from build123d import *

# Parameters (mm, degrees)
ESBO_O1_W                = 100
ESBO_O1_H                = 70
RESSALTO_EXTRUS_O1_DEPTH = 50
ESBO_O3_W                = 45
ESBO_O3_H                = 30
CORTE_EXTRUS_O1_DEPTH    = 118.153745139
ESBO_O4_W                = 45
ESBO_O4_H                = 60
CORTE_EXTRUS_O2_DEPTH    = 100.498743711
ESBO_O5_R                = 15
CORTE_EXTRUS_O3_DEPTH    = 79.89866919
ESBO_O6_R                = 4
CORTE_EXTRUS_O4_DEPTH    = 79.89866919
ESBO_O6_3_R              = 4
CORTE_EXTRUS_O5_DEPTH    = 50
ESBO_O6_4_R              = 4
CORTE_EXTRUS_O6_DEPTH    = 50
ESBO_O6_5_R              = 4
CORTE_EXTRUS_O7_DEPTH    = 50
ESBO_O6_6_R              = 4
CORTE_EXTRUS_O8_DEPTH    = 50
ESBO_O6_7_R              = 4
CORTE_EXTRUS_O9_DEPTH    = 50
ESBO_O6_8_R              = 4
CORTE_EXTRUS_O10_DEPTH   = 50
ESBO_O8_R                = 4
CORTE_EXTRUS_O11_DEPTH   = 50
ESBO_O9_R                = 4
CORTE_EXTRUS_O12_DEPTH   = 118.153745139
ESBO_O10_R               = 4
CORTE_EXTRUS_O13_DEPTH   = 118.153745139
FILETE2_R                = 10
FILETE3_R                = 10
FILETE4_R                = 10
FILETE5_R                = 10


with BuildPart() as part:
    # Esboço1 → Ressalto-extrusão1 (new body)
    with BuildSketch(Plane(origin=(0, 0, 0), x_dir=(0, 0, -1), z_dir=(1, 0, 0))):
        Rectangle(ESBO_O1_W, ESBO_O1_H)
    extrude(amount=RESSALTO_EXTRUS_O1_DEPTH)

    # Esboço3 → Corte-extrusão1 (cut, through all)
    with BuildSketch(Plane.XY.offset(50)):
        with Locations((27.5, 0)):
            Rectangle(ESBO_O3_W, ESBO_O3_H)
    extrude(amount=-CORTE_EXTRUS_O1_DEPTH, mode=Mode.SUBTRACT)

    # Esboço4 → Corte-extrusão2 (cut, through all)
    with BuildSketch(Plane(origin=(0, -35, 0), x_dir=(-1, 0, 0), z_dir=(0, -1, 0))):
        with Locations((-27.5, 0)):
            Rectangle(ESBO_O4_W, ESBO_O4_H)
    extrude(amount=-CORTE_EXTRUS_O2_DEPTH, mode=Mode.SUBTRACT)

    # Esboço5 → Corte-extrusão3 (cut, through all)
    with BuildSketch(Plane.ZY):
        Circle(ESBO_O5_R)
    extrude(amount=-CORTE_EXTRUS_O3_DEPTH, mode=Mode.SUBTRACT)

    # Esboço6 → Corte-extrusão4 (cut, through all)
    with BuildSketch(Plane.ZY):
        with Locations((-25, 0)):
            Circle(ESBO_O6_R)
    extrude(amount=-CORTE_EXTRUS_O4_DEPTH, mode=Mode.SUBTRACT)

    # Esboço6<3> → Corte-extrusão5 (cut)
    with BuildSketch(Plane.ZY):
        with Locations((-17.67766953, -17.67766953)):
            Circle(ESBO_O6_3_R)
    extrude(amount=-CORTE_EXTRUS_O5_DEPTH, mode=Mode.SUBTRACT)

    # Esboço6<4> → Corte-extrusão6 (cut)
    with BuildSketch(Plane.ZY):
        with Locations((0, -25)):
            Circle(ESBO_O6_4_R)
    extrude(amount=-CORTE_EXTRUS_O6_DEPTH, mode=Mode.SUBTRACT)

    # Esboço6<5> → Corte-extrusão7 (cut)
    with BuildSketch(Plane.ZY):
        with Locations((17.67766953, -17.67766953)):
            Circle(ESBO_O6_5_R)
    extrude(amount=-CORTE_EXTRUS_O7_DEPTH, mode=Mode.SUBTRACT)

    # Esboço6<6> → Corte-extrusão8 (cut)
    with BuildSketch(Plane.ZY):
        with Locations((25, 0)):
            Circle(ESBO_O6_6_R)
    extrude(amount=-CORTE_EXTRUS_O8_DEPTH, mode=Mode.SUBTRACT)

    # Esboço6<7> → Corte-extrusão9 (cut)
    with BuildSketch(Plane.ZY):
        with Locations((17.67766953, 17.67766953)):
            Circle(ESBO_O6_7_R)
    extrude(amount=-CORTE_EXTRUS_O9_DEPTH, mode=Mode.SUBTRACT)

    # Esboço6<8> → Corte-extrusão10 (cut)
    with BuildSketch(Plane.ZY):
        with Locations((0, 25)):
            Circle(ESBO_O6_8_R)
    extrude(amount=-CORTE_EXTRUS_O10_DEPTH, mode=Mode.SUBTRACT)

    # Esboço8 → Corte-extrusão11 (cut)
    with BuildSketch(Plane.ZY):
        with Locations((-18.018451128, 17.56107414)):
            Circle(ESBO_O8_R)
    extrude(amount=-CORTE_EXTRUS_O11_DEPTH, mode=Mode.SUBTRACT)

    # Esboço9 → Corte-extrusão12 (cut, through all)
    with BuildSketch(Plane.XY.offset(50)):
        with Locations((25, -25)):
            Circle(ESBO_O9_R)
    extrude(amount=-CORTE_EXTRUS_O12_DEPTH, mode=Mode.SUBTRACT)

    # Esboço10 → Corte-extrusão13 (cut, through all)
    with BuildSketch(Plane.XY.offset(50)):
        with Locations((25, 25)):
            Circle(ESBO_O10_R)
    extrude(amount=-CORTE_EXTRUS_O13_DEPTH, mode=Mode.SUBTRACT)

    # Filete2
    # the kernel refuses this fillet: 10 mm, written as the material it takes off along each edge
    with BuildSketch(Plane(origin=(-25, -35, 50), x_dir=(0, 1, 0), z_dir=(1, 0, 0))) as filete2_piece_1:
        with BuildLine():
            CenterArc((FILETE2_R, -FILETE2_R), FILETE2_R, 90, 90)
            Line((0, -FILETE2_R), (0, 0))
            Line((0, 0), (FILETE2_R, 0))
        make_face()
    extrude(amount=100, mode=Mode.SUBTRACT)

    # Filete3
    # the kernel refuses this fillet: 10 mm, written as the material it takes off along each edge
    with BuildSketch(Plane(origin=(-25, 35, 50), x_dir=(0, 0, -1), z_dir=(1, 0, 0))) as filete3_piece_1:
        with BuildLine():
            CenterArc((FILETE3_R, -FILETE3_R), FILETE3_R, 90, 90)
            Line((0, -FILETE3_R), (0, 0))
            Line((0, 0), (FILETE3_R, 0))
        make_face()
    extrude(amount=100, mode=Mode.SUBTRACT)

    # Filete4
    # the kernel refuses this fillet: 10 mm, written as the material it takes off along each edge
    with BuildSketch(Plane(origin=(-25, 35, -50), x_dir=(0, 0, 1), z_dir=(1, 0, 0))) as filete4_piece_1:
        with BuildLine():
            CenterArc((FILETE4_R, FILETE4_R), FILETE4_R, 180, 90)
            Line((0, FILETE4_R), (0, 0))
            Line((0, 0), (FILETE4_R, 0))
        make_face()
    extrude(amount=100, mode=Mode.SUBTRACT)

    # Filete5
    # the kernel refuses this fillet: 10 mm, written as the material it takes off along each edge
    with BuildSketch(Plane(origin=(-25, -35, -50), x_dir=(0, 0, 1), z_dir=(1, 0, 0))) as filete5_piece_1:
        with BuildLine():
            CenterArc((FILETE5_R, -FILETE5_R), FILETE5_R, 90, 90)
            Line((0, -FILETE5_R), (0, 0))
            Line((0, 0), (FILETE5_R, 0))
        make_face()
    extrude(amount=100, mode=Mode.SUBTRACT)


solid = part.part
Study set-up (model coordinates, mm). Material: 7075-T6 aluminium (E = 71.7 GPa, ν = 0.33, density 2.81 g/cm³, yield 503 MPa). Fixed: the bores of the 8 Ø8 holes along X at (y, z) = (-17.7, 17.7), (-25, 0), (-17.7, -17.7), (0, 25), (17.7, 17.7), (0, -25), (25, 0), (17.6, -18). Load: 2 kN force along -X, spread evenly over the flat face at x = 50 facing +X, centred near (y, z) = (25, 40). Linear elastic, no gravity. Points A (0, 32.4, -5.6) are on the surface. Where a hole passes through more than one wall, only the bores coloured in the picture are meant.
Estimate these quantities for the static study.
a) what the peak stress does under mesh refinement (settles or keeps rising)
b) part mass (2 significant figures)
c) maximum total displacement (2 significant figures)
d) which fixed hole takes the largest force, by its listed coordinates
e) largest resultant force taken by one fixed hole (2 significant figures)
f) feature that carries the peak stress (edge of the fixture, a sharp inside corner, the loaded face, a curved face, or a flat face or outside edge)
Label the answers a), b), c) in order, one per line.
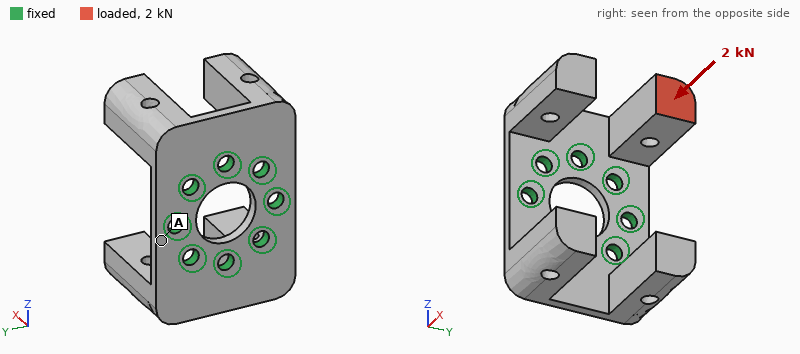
a) keeps rising
b) 260 g
c) 0.58 mm
d) (17.7, 17.7)
e) 1.7 kN
f) edge of the fixture
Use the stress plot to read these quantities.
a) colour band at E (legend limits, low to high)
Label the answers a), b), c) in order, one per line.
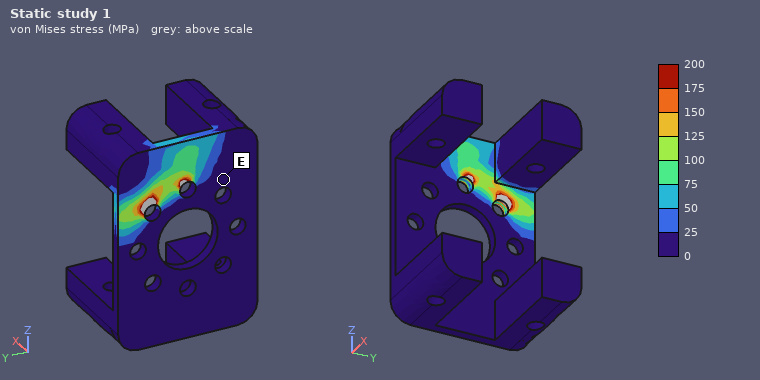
a) 0 to 25 MPa
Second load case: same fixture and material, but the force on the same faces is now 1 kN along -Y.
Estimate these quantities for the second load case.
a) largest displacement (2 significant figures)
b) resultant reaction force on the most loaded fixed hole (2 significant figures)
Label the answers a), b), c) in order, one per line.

a) 0.64 mm
b) 1.7 kN
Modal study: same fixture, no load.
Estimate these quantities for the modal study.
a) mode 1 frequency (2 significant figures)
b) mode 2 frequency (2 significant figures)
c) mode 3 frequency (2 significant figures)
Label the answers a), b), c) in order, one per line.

a) 1100 Hz
b) 1100 Hz
c) 1200 Hz
